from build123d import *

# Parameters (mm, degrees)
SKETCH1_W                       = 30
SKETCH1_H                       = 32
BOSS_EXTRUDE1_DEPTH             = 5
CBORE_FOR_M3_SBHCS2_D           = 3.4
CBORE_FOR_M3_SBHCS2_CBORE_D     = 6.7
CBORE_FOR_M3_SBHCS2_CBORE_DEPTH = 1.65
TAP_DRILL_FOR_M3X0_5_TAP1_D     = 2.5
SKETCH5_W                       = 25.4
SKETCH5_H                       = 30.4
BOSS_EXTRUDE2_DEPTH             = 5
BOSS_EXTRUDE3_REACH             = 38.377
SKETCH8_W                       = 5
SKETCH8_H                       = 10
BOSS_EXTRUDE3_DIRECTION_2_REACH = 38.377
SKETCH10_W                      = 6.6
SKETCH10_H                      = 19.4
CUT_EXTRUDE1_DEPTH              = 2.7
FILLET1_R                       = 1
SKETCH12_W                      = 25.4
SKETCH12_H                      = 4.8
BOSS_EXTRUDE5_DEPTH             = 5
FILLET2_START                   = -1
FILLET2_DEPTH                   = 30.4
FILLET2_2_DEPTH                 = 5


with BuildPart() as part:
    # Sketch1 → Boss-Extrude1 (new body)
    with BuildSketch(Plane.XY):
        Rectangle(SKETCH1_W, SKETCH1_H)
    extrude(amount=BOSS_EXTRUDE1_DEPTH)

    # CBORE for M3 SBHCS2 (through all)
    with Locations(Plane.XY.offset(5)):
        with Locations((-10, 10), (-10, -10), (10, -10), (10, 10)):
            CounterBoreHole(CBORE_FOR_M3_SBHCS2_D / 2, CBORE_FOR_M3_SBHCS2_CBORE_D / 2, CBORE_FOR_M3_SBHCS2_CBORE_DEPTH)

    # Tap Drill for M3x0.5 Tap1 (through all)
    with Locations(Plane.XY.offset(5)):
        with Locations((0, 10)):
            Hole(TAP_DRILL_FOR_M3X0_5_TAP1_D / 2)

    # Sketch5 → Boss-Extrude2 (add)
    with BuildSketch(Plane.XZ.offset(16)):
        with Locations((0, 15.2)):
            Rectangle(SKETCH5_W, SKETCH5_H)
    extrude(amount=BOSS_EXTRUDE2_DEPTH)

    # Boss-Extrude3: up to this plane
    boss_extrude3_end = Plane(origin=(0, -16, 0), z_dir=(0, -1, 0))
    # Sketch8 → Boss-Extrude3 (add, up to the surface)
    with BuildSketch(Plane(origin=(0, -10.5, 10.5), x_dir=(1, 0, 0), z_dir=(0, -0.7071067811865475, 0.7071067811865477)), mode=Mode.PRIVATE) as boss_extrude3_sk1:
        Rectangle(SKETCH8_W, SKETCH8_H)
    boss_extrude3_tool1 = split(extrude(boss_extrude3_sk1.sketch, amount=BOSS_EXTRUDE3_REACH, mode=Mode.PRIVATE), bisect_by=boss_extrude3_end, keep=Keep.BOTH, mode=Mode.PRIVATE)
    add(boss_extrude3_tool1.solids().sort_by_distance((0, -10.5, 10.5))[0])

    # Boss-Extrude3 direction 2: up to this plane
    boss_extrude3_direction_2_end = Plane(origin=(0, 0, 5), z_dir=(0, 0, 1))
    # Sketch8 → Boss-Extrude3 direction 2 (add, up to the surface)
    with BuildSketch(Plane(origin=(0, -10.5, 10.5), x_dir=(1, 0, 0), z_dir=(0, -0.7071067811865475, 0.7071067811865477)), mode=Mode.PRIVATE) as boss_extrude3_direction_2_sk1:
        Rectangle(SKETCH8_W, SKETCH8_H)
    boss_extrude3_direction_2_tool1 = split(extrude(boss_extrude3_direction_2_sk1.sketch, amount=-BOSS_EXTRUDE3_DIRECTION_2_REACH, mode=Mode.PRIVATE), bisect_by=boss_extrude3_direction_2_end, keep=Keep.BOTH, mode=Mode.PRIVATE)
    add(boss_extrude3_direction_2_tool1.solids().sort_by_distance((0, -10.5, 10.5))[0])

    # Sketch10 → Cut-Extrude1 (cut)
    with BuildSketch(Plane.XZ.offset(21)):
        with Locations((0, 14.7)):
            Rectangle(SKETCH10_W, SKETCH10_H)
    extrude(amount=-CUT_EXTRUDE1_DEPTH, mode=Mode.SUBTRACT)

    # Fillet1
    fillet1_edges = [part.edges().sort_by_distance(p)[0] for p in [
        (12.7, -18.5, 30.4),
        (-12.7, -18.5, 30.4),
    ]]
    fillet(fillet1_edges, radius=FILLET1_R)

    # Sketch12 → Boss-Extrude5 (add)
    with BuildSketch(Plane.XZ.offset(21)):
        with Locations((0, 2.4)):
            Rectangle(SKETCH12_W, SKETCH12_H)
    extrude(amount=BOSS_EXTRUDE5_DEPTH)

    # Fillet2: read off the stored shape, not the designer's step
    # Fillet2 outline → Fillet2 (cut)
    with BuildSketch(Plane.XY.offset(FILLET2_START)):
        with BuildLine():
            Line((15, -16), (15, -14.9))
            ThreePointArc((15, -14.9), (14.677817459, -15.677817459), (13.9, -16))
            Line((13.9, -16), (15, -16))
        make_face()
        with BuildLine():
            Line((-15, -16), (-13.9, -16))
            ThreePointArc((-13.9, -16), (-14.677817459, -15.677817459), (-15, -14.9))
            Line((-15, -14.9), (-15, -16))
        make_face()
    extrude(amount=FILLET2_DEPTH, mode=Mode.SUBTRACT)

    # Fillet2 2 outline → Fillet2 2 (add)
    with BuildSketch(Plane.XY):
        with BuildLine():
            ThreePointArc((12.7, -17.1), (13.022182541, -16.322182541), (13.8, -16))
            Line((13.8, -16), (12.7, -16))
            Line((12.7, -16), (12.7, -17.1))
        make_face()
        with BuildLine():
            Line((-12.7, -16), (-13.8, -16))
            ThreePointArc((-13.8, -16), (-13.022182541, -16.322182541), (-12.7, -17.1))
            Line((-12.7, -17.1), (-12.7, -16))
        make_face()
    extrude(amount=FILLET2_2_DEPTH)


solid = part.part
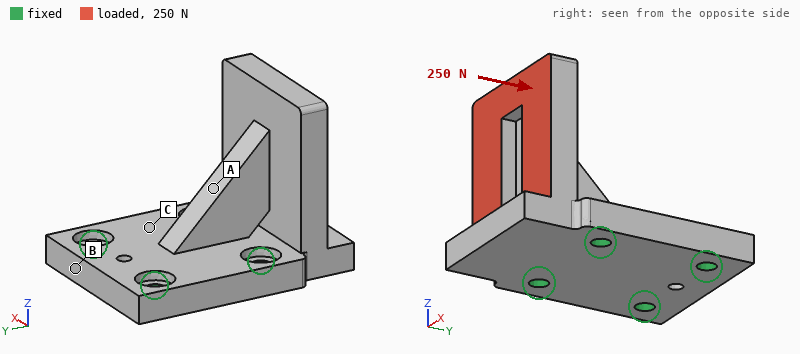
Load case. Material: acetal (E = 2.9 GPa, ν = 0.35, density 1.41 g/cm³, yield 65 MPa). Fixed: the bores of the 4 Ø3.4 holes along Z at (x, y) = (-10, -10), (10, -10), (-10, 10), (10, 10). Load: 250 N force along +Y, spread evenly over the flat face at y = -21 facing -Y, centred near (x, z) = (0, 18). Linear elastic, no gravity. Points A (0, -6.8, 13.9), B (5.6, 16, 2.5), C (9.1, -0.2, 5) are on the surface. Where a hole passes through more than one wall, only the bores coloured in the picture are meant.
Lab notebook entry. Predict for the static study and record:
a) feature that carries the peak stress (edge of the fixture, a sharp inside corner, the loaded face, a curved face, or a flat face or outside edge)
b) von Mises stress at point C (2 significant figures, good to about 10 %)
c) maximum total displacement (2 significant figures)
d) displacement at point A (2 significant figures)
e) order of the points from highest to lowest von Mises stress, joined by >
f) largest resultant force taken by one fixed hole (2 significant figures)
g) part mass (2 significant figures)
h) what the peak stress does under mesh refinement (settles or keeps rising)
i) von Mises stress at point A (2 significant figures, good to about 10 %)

edge of the fixture
4.7 MPa
0.53 mm
0.14 mm
A > C > B
140 N
13 g
keeps rising
13 MPa
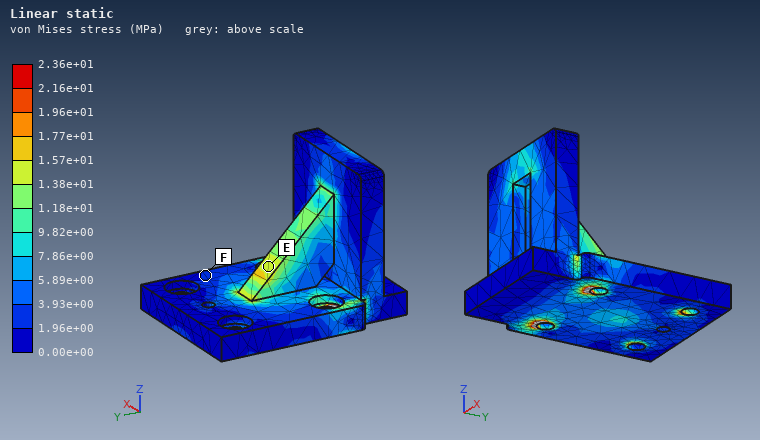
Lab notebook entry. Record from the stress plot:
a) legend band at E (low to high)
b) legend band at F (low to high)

1.38e+01 to 1.57e+01 MPa
1.96e+00 to 3.93e+00 MPa
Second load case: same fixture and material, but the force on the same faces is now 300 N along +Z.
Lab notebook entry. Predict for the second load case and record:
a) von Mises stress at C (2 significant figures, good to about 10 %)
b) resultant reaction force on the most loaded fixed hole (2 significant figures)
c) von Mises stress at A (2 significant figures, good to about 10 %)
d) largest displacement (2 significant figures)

3.4 MPa
220 N
6.7 MPa
0.39 mm
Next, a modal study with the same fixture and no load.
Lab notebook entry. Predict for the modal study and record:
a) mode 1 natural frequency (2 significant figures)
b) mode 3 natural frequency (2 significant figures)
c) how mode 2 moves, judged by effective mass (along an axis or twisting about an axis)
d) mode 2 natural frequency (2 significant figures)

1900 Hz
3400 Hz
along X
2600 Hz
